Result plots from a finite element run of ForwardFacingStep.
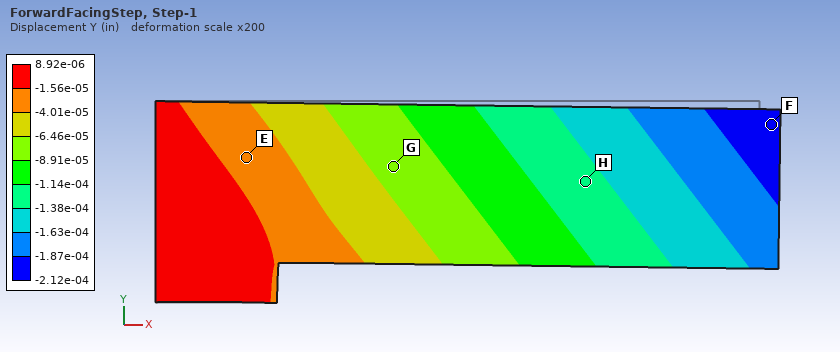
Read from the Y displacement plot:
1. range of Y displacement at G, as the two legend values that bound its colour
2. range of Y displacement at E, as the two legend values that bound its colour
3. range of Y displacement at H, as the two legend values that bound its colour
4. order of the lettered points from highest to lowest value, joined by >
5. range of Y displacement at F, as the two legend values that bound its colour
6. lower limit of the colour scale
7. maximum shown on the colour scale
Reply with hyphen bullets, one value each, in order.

- -8.91e-05 to -6.46e-05 in
- -4.01e-05 to -1.56e-05 in
- -1.38e-04 to -1.14e-04 in
- E > G > H > F
- -2.12e-04 to -1.87e-04 in
- -2.12e-04 in
- 8.92e-06 in
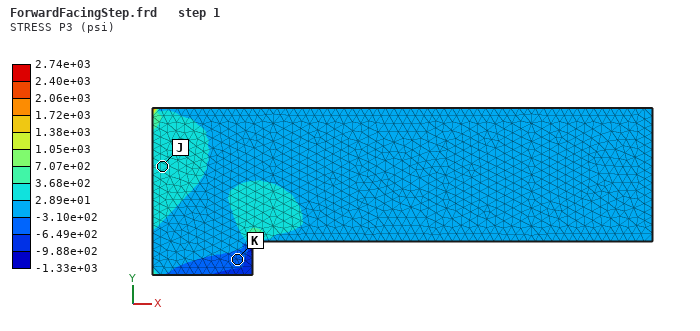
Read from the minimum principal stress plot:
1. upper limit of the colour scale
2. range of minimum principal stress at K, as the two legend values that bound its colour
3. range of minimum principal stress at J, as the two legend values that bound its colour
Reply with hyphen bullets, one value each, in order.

- 2.74e+03 psi
- -6.49e+02 to -3.10e+02 psi
- 2.89e+01 to 3.68e+02 psi
